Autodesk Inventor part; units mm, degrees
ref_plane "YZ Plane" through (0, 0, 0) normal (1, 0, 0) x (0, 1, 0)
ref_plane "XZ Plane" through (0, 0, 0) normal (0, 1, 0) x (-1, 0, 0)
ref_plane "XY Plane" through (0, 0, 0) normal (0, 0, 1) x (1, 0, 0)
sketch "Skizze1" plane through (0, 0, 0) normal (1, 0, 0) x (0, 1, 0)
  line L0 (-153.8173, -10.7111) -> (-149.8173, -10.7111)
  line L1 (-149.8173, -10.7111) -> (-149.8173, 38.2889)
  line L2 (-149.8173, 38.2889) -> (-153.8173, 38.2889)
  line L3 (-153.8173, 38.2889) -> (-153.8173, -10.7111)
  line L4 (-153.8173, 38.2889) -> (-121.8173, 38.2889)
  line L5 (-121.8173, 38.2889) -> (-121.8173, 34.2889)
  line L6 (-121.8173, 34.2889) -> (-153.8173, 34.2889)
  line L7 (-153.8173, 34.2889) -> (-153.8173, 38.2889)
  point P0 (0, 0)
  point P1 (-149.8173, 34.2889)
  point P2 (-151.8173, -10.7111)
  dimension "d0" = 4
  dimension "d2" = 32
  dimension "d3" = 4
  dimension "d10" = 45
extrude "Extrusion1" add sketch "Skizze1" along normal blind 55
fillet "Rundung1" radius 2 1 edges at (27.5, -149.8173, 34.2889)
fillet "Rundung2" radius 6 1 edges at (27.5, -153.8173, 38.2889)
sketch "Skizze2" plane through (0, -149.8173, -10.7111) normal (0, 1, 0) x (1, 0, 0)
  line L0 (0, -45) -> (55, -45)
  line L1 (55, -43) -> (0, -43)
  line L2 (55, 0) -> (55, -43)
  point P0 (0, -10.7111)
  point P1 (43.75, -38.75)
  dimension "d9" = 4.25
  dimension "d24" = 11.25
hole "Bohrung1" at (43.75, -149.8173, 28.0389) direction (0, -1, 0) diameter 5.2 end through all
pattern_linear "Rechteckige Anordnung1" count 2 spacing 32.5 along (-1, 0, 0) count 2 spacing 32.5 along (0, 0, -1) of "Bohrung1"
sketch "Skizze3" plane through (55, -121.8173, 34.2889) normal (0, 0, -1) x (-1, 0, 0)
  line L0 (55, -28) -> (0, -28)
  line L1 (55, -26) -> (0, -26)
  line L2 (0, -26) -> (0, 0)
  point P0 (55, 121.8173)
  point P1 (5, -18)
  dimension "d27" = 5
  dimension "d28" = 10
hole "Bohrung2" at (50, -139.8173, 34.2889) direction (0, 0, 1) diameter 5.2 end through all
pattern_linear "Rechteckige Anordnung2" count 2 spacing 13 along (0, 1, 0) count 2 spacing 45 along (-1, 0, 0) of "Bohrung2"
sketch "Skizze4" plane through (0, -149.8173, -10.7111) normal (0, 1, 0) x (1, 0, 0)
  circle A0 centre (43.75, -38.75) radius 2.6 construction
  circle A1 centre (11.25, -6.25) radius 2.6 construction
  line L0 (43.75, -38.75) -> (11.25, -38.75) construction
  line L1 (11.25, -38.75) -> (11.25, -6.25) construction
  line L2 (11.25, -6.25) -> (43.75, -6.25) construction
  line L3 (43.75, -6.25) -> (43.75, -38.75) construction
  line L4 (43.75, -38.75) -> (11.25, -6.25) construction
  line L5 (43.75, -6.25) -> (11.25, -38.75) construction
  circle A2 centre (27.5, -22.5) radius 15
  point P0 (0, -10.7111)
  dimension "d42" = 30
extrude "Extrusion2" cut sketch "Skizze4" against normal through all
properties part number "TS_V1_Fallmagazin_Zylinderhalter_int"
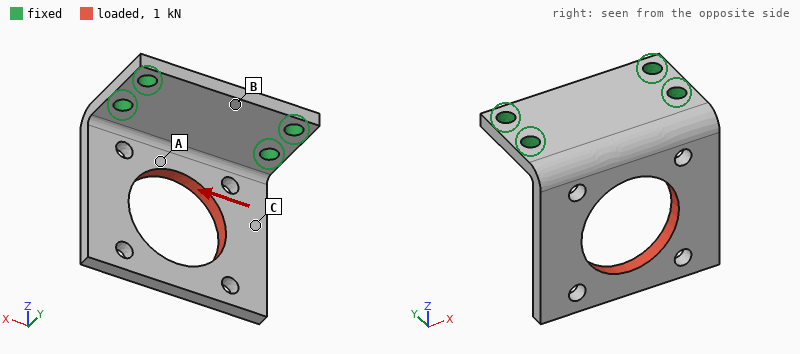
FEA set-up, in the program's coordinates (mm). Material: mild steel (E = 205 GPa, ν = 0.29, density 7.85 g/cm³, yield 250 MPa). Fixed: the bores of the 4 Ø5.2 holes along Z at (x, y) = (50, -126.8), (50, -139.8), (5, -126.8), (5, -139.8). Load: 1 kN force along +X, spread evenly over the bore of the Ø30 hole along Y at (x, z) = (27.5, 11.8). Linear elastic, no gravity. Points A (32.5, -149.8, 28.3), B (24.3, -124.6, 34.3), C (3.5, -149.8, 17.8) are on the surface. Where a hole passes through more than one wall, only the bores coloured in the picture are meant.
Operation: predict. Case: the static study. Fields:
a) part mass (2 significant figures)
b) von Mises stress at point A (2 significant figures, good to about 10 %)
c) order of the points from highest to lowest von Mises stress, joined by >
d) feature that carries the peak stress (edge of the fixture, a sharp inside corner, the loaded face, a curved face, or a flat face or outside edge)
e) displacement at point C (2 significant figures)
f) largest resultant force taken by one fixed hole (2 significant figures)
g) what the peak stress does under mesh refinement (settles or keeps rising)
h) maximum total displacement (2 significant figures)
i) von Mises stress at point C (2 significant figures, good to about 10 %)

100 g
37 MPa
A > C > B
edge of the fixture
21 µm
740 N
keeps rising
41 µm
22 MPa
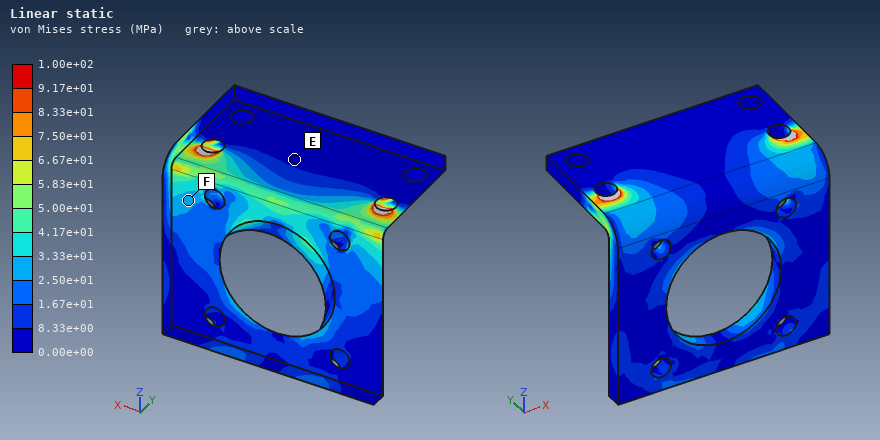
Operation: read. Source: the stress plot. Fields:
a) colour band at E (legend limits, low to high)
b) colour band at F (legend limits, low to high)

0.00e+00 to 8.33e+00 MPa
2.50e+01 to 3.33e+01 MPa
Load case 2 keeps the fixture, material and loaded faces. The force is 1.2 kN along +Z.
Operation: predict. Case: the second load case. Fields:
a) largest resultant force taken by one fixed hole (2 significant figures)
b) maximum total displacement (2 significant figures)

730 N
76 µm
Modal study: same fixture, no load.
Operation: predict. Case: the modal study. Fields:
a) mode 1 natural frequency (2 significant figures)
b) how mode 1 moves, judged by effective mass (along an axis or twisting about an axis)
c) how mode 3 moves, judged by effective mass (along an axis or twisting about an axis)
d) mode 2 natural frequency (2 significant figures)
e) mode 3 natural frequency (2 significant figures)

1100 Hz
along Y
along X
2300 Hz
4500 Hz
